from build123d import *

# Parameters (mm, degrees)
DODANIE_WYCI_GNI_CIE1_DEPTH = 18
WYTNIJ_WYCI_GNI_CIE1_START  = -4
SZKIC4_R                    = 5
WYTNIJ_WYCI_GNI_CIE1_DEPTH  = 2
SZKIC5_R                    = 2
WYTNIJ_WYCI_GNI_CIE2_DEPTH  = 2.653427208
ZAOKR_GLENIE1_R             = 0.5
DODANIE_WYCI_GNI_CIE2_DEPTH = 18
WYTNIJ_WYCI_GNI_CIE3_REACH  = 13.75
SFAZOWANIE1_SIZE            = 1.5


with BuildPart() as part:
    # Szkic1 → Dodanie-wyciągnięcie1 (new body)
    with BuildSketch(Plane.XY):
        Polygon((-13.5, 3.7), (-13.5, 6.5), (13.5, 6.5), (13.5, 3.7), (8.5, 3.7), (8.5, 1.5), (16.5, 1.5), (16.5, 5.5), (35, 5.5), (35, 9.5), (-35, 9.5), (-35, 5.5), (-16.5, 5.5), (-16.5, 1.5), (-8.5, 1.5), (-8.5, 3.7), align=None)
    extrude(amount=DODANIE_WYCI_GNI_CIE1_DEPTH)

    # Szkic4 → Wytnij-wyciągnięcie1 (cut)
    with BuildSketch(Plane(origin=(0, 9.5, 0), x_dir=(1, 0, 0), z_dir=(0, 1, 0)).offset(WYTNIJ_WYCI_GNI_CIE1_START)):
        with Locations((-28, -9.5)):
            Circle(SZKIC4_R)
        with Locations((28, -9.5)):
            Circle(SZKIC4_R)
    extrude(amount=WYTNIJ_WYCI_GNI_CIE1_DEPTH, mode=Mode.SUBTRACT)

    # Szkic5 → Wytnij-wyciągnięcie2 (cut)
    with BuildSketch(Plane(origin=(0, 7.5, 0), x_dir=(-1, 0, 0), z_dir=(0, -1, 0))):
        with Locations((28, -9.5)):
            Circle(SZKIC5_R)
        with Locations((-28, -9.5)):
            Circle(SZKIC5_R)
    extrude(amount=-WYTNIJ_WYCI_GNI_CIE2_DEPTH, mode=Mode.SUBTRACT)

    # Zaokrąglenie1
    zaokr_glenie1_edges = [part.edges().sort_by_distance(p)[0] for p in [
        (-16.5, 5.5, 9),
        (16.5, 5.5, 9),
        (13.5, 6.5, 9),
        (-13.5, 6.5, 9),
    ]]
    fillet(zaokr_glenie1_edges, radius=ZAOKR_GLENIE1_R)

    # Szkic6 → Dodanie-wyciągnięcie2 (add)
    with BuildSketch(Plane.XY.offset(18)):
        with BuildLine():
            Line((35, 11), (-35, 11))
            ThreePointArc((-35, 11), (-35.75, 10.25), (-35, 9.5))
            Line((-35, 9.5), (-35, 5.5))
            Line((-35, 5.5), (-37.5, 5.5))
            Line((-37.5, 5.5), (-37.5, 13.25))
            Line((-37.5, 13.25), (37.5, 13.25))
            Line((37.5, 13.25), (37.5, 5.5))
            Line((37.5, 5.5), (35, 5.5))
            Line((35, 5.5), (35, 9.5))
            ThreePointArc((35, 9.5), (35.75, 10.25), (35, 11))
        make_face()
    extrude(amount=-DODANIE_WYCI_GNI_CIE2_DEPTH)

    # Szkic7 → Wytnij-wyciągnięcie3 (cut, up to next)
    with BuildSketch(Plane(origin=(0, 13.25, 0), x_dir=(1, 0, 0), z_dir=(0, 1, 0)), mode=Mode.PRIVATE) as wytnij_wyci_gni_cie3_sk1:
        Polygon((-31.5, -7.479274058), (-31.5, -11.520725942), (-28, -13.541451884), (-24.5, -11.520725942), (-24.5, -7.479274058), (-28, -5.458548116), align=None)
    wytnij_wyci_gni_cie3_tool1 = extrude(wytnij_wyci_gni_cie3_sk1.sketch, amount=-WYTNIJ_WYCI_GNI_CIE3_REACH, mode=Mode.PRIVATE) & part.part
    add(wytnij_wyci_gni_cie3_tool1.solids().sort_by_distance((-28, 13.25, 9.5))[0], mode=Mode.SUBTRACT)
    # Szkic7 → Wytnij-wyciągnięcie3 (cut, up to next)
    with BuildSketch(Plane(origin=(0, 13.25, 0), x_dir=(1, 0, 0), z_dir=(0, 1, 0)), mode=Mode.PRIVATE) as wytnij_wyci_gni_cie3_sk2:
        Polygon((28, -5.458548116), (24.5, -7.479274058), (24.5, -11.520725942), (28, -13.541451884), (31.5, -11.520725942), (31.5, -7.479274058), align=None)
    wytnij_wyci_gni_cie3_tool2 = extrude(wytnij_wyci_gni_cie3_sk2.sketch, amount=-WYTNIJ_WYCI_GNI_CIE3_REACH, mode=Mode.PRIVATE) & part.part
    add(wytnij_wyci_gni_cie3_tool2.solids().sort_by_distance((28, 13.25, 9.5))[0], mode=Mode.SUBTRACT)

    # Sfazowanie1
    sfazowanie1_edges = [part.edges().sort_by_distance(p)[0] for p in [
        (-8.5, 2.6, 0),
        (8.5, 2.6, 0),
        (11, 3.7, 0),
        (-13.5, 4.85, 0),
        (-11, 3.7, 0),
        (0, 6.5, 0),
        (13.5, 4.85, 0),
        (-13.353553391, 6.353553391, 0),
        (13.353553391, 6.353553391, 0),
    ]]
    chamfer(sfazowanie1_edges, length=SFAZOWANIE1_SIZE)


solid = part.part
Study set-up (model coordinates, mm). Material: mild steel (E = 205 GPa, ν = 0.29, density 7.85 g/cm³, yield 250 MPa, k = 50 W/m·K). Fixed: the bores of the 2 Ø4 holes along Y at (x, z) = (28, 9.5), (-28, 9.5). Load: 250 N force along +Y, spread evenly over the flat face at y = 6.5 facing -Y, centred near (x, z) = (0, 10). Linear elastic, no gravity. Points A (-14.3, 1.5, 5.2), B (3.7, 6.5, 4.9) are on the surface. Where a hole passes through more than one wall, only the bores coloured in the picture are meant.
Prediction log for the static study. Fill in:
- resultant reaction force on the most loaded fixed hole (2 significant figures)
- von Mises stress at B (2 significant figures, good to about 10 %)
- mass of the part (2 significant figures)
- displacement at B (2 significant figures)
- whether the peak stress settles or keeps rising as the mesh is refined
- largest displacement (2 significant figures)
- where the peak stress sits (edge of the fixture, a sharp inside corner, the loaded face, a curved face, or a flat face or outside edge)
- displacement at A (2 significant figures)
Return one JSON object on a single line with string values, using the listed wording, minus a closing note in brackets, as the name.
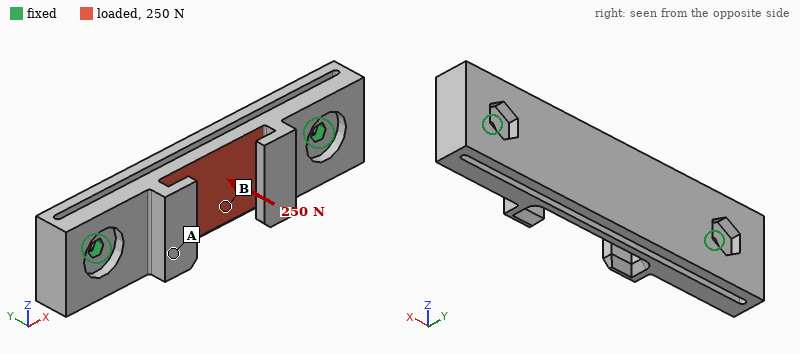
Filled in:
{"resultant reaction force on the most loaded fixed hole": "130 N", "von Mises stress at B": "36 MPa", "mass of the part": "65 g", "displacement at B": "22 µm", "whether the peak stress settles or keeps rising as the mesh is refined": "keeps rising", "largest displacement": "25 µm", "where the peak stress sits": "edge of the fixture", "displacement at A": "15 µm"}
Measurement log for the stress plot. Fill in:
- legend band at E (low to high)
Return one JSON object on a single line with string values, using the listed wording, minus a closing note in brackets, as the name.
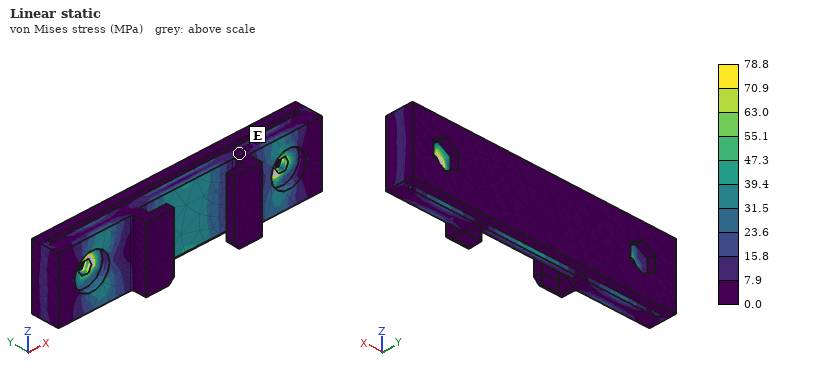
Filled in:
{"legend band at E": "0.0 to 7.9 MPa"}
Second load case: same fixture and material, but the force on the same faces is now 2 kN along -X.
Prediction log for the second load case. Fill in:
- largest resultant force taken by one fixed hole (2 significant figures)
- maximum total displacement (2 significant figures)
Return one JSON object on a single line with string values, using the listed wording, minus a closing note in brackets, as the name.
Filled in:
{"largest resultant force taken by one fixed hole": "1.0 kN", "maximum total displacement": "3.1 µm"}
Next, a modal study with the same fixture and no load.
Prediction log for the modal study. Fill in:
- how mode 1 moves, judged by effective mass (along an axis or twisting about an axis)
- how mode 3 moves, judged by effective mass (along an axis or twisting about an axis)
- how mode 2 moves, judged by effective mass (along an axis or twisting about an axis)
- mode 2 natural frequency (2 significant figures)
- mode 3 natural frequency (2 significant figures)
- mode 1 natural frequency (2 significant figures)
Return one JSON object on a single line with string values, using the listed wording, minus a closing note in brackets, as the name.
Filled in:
{"how mode 1 moves, judged by effective mass": "along Y", "how mode 3 moves, judged by effective mass": "twisting about X", "how mode 2 moves, judged by effective mass": "along Y", "mode 2 natural frequency": "4200 Hz", "mode 3 natural frequency": "4800 Hz", "mode 1 natural frequency": "1900 Hz"}
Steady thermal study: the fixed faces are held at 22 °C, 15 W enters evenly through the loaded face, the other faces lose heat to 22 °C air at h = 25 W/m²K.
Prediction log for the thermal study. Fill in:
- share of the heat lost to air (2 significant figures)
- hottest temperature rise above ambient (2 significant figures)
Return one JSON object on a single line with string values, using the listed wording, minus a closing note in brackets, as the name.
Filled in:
{"share of the heat lost to air": "17 %", "hottest temperature rise above ambient": "55 K"}
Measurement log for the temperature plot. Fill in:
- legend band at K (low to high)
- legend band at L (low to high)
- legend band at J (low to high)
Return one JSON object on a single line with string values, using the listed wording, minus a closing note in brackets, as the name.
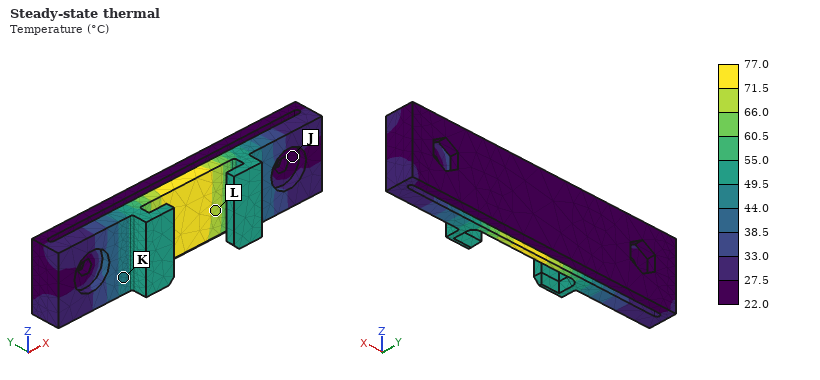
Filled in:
{"legend band at K": "44.0 to 49.5 °C", "legend band at L": "66.0 to 71.5 °C", "legend band at J": "22.0 to 27.5 °C"}
